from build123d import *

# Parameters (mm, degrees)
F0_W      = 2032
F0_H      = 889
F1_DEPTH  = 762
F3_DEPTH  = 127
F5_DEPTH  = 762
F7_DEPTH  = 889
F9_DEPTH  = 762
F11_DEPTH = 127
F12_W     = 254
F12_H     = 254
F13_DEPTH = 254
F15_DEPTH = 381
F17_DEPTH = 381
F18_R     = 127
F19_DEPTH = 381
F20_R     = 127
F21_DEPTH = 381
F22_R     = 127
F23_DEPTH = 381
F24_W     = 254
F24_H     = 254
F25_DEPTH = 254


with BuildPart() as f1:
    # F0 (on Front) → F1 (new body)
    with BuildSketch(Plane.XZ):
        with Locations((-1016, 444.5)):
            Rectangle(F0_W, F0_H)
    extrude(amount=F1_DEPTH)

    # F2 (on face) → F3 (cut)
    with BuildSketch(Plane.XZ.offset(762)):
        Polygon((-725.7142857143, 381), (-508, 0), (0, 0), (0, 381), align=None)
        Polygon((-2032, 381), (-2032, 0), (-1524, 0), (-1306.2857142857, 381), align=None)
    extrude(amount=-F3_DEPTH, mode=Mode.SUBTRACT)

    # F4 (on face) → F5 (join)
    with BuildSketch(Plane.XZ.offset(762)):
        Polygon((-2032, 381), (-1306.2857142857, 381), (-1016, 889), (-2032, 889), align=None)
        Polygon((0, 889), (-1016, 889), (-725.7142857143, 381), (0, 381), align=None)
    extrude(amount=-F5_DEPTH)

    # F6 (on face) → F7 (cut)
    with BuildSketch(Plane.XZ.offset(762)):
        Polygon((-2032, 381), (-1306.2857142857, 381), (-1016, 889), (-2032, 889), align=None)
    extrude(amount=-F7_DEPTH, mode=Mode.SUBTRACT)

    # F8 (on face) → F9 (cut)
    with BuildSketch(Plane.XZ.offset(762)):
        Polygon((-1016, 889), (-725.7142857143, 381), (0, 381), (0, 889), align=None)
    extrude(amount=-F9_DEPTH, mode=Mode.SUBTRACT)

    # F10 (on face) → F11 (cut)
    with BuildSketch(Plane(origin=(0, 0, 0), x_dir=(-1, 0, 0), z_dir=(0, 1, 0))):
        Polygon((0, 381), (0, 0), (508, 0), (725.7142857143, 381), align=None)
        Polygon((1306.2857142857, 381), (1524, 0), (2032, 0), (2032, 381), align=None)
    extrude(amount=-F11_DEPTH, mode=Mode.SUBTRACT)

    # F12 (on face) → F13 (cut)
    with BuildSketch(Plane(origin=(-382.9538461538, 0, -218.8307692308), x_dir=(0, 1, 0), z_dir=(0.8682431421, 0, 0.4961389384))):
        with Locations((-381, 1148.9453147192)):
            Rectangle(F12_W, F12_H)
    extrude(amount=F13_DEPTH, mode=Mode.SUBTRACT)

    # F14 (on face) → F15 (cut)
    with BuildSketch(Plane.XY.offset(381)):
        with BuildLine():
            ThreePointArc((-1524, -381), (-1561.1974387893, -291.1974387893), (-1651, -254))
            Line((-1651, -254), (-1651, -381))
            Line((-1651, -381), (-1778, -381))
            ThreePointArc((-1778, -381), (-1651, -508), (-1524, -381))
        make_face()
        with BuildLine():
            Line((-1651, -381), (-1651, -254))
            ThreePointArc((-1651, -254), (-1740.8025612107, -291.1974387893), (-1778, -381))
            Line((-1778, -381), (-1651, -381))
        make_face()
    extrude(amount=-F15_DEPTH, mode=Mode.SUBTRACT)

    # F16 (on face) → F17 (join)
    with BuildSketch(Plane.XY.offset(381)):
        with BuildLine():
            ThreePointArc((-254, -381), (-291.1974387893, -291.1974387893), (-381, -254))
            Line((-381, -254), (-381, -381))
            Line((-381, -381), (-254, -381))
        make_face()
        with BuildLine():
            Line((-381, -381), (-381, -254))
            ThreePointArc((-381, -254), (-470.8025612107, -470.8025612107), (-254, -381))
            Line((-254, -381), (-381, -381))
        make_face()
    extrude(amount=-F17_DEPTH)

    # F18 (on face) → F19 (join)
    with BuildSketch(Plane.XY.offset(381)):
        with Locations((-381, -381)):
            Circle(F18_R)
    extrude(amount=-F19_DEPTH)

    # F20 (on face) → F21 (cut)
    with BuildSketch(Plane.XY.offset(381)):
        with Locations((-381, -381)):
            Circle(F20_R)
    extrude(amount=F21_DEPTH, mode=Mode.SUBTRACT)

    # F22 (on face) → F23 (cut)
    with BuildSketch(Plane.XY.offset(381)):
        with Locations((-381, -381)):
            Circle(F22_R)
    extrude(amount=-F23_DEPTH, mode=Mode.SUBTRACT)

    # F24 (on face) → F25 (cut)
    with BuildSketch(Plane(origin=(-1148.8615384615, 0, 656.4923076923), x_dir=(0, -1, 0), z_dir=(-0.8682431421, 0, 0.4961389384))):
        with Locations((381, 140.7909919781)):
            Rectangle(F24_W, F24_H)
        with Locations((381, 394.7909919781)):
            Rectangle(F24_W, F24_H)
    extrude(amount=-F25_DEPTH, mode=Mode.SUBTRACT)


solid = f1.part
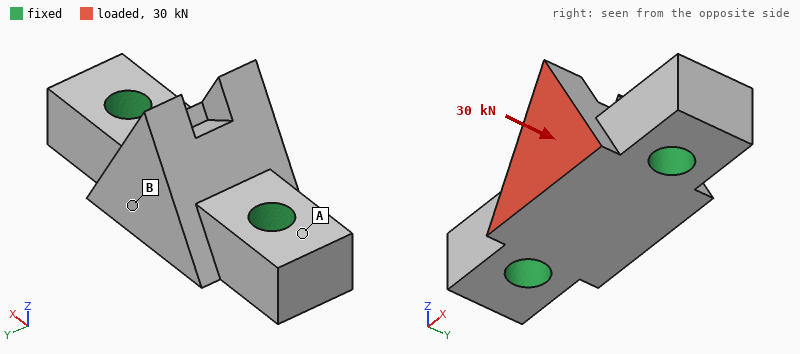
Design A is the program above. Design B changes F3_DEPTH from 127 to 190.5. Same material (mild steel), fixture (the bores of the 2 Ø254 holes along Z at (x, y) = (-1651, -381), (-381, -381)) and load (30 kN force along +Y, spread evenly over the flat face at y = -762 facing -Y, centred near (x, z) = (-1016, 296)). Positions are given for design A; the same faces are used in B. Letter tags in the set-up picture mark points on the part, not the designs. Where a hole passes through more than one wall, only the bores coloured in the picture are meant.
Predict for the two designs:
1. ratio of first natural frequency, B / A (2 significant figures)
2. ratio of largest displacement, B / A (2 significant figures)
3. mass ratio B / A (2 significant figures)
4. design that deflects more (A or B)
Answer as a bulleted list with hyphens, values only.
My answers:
- 0.92
- 1.1
- 0.94
- B
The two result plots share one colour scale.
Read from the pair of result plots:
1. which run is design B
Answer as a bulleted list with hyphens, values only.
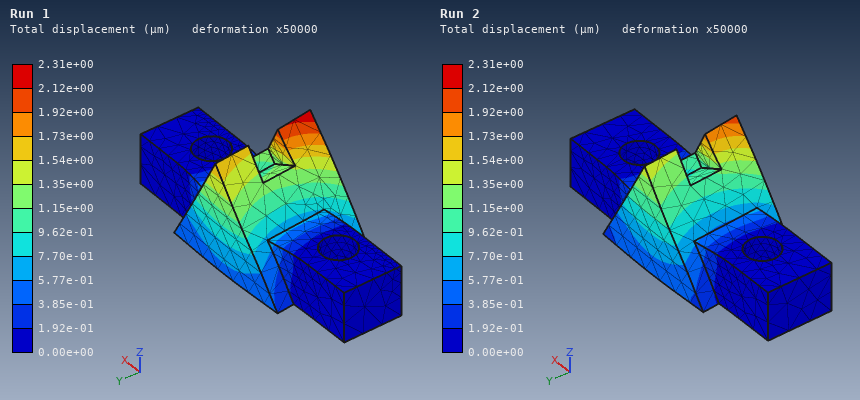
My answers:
- Run 1
